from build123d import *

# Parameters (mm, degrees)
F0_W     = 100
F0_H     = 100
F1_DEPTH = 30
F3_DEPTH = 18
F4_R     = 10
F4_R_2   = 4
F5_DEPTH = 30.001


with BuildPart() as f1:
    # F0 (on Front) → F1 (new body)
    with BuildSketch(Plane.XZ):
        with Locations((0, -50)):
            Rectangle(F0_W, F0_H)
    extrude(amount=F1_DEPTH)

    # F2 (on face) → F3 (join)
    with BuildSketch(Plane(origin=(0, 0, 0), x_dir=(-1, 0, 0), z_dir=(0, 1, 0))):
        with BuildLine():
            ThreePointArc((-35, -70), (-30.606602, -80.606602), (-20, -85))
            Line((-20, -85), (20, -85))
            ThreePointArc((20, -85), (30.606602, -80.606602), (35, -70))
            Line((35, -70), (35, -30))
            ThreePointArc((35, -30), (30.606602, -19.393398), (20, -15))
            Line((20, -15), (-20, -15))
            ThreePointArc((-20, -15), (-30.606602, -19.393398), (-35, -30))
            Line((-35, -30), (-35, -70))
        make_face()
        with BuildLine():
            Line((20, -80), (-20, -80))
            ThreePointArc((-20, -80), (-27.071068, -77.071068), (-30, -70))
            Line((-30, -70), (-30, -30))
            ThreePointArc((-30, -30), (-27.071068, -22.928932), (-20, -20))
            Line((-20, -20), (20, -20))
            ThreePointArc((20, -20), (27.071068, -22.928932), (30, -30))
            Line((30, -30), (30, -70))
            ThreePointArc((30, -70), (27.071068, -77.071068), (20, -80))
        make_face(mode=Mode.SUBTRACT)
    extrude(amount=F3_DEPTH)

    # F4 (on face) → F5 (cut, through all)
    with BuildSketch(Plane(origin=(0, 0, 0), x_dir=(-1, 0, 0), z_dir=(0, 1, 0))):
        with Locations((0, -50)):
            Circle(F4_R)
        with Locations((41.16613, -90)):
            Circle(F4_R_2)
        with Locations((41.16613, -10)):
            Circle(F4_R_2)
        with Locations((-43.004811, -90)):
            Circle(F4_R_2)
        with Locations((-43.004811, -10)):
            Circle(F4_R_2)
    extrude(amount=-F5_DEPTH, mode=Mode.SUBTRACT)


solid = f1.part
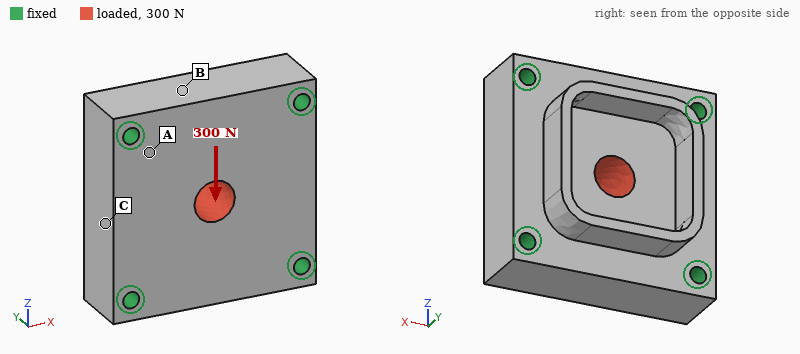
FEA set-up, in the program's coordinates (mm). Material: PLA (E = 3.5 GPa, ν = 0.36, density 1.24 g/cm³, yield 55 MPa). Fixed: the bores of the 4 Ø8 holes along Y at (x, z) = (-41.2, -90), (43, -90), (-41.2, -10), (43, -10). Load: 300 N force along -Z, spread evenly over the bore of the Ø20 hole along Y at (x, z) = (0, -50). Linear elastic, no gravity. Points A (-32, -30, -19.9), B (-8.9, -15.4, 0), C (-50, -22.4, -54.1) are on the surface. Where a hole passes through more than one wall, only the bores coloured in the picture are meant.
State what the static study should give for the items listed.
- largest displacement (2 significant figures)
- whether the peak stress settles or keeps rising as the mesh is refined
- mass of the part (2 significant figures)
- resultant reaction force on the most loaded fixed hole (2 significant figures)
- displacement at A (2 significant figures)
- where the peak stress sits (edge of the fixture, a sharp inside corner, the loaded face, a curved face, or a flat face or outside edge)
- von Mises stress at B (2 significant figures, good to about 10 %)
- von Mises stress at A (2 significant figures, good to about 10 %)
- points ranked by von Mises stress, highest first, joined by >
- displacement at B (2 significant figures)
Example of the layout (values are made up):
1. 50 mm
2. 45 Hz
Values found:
1. 2.3 µm
2. keeps rising
3. 380 g
4. 87 N
5. 0.57 µm
6. edge of the fixture
7. 0.076 MPa
8. 0.14 MPa
9. A > B > C
10. 1.5 µm
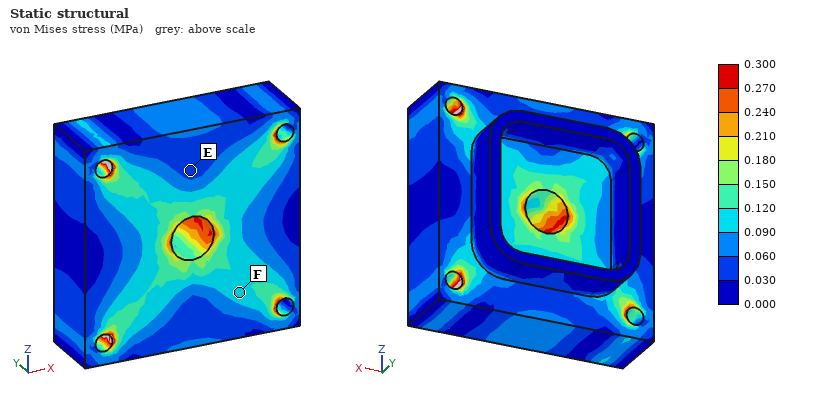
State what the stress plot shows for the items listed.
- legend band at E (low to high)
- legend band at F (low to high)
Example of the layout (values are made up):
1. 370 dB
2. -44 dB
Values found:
1. 0.030 to 0.060 MPa
2. 0.090 to 0.120 MPa
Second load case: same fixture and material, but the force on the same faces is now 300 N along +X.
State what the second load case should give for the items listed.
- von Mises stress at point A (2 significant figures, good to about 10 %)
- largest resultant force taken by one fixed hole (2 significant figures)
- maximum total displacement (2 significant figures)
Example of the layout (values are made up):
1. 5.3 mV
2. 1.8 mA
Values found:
1. 0.13 MPa
2. 86 N
3. 2.2 µm
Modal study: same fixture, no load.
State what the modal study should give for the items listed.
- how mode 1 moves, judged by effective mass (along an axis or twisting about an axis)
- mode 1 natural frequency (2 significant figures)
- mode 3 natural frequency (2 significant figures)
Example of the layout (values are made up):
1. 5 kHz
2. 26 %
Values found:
1. along Y
2. 3300 Hz
3. 4200 Hz
